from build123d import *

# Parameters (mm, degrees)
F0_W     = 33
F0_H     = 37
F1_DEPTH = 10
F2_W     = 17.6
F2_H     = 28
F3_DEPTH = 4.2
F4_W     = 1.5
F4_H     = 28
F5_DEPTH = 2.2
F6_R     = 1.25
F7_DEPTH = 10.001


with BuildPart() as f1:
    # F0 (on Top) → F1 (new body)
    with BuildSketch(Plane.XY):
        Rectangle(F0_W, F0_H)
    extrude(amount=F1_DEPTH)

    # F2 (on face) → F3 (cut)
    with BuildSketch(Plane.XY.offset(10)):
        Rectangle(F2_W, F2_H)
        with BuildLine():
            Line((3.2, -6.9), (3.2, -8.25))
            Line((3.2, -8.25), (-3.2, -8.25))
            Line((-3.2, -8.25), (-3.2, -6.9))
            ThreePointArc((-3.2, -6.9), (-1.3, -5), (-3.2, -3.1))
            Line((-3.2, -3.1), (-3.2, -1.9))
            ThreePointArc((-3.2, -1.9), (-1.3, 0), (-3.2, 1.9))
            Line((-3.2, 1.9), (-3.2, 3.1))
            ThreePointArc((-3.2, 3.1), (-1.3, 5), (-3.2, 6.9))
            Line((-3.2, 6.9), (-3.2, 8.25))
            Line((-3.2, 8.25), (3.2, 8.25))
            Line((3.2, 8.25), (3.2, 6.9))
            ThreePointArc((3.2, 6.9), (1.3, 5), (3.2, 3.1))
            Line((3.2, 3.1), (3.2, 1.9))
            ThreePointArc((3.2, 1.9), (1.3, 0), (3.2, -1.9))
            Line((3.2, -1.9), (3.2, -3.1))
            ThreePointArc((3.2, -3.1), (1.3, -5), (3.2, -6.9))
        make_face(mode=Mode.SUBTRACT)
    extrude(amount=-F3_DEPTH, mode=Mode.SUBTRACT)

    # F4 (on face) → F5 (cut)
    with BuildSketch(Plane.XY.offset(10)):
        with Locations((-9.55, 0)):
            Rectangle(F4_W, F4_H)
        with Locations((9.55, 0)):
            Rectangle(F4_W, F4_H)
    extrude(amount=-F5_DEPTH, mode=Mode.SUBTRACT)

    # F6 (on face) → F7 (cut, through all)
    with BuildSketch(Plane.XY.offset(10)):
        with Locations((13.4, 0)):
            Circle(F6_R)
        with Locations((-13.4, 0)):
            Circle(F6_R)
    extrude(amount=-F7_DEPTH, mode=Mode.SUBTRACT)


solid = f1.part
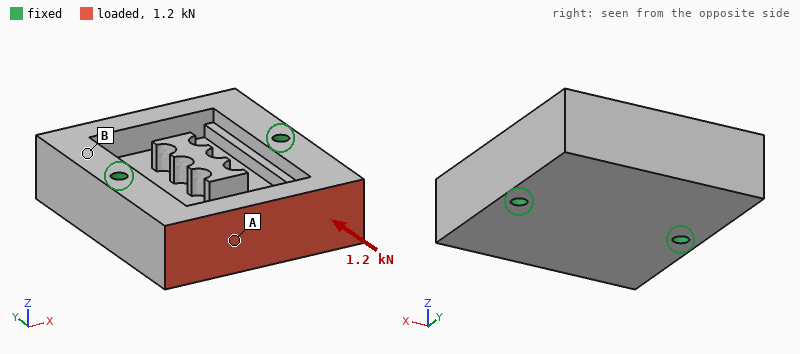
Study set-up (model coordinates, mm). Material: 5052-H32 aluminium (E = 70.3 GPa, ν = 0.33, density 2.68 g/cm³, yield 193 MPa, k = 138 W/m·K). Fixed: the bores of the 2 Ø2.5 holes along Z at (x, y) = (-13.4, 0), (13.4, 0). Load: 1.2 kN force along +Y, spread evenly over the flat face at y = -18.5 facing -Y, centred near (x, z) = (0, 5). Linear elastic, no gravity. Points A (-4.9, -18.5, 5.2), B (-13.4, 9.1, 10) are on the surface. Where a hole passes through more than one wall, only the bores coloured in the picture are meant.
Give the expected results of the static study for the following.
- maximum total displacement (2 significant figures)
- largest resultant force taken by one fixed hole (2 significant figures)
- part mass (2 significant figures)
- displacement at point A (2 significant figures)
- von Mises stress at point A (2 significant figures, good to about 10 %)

4.7 µm
610 N
27 g
2.8 µm
7.2 MPa
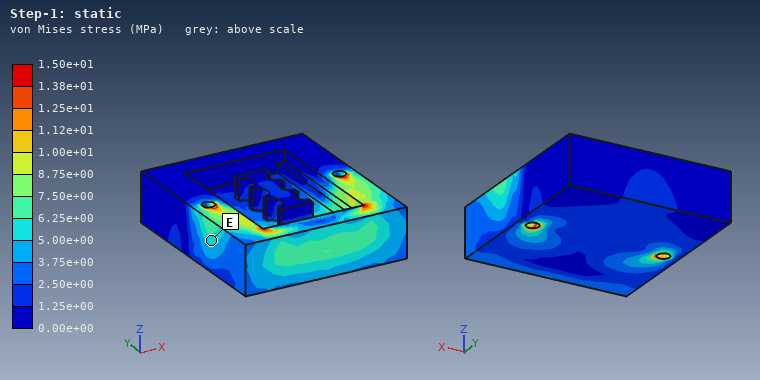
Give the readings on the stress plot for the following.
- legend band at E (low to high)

5.00e+00 to 6.25e+00 MPa
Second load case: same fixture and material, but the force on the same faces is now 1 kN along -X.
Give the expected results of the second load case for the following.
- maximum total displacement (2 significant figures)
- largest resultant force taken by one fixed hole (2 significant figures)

7.9 µm
820 N
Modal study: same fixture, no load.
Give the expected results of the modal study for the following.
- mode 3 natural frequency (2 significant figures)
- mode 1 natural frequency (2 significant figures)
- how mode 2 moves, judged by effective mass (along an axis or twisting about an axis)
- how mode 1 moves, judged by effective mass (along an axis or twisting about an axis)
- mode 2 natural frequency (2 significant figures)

22 kHz
13 kHz
along Z
twisting about X
16 kHz
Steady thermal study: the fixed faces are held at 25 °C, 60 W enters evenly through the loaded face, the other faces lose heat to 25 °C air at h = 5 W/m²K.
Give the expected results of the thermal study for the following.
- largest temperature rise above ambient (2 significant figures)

38 K
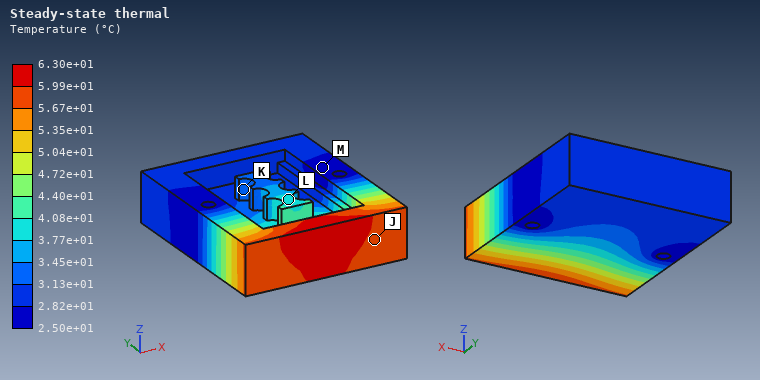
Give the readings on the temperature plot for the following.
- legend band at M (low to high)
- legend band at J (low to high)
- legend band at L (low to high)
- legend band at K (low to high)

2.50e+01 to 2.82e+01 °C
5.67e+01 to 5.99e+01 °C
3.77e+01 to 4.08e+01 °C
3.13e+01 to 3.45e+01 °C
